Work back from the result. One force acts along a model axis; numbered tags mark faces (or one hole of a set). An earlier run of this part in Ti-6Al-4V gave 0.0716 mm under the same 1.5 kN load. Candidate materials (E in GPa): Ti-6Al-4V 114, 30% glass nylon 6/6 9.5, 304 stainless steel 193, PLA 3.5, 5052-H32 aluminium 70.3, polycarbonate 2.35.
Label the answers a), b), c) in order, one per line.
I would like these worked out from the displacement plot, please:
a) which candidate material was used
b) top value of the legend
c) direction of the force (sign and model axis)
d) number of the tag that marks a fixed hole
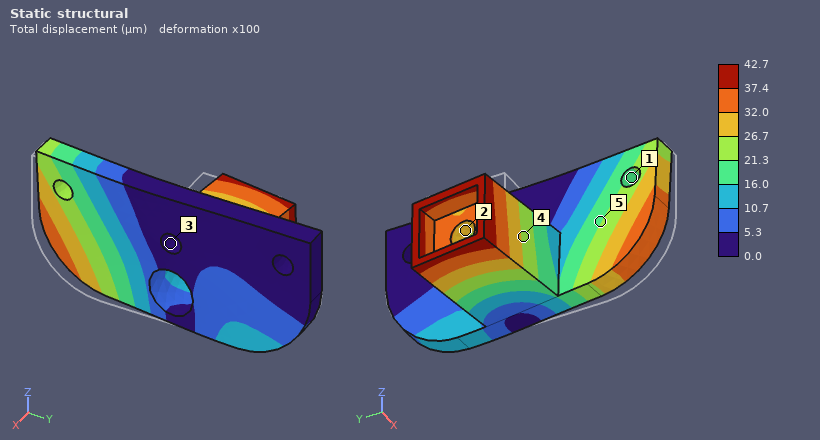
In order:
a) 304 stainless steel
b) 42.7 µm
c) +Y
d) 3
